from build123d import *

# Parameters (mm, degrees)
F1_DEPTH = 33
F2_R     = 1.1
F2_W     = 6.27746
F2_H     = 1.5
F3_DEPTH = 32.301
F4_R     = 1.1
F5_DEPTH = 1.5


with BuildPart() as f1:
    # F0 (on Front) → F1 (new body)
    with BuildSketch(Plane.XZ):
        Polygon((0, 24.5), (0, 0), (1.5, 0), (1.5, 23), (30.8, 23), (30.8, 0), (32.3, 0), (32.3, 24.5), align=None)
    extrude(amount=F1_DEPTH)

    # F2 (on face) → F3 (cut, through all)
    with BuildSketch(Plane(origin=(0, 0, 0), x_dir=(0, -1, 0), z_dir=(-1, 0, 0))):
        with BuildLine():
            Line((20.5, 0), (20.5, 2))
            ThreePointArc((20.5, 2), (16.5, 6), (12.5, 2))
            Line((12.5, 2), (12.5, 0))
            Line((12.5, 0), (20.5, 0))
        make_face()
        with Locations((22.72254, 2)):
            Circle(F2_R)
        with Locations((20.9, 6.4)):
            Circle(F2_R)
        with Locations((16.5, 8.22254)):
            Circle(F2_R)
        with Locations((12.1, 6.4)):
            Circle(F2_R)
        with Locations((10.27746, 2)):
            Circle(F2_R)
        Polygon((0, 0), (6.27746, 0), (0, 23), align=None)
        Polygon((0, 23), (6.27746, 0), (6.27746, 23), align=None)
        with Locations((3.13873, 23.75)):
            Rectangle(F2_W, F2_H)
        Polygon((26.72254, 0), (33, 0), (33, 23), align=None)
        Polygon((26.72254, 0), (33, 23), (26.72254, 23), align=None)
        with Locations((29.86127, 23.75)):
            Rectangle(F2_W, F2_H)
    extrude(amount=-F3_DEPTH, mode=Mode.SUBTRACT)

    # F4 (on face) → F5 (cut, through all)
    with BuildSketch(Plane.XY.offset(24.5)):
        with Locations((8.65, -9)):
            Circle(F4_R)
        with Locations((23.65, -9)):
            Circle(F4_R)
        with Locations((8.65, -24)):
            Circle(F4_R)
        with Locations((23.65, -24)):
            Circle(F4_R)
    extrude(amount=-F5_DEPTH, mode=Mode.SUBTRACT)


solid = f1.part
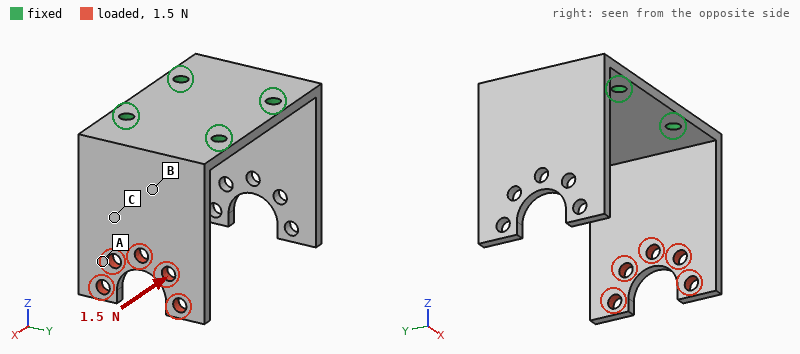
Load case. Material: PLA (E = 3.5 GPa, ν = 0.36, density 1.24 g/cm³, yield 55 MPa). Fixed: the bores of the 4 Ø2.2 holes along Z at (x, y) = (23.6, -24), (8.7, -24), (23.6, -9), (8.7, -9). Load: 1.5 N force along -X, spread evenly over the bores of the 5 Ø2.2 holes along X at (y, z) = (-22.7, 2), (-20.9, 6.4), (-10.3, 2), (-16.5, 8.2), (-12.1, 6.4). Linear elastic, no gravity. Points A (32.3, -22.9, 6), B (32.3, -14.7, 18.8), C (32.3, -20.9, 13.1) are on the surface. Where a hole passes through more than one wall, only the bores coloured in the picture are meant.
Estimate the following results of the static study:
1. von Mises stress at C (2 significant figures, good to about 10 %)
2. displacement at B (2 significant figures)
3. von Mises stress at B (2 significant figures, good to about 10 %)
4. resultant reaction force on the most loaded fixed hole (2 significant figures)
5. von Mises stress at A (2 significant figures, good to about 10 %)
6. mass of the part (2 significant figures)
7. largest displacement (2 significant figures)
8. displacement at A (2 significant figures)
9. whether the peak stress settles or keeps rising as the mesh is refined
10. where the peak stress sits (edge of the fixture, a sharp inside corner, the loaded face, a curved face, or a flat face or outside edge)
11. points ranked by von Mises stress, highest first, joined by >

1.5 MPa
0.078 mm
2.3 MPa
0.71 N
0.56 MPa
2.7 g
0.43 mm
0.30 mm
keeps rising
edge of the fixture
B > C > A
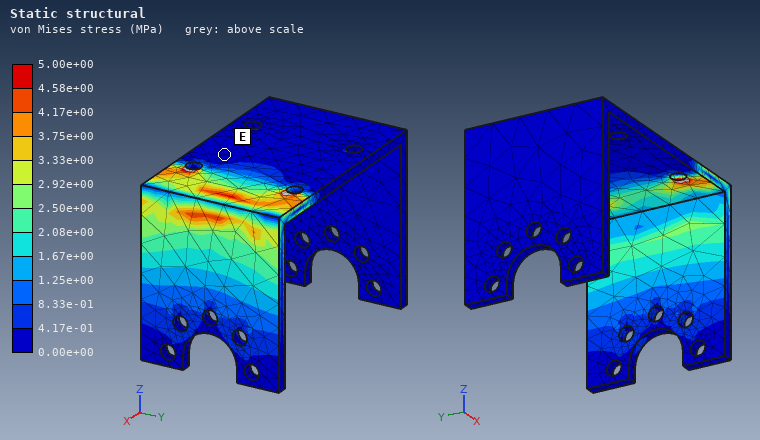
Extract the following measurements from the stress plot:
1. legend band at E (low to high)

0.00e+00 to 4.17e-01 MPa
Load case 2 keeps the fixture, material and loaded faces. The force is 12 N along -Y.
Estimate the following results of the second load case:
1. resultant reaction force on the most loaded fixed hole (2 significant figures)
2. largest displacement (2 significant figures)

17 N
0.44 mm
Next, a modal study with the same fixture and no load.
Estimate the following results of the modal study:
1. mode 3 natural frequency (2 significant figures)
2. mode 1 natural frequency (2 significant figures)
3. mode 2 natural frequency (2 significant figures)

1400 Hz
590 Hz
590 Hz
